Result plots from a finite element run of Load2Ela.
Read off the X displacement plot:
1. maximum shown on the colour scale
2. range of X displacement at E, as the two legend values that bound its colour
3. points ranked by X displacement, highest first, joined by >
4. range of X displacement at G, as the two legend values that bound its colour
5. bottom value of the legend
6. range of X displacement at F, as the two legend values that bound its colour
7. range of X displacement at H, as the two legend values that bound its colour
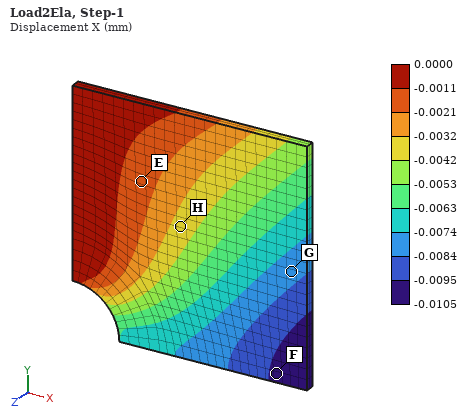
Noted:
0.0000 mm
-0.0021 to -0.0011 mm
E > H > G > F
-0.0084 to -0.0074 mm
-0.0105 mm
-0.0105 to -0.0095 mm
-0.0042 to -0.0032 mm
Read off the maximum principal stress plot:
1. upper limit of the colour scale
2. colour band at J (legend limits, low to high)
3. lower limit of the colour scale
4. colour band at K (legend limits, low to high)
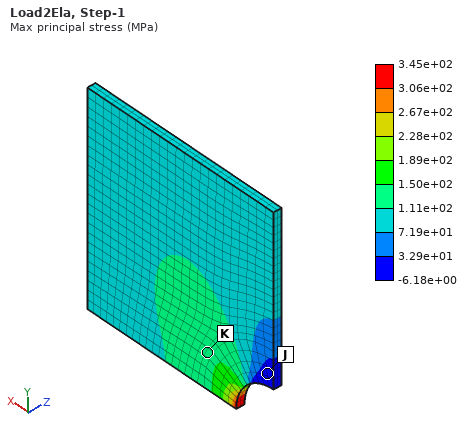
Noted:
3.45e+02 MPa
-6.18e+00 to 3.29e+01 MPa
-6.18e+00 MPa
1.11e+02 to 1.50e+02 MPa
